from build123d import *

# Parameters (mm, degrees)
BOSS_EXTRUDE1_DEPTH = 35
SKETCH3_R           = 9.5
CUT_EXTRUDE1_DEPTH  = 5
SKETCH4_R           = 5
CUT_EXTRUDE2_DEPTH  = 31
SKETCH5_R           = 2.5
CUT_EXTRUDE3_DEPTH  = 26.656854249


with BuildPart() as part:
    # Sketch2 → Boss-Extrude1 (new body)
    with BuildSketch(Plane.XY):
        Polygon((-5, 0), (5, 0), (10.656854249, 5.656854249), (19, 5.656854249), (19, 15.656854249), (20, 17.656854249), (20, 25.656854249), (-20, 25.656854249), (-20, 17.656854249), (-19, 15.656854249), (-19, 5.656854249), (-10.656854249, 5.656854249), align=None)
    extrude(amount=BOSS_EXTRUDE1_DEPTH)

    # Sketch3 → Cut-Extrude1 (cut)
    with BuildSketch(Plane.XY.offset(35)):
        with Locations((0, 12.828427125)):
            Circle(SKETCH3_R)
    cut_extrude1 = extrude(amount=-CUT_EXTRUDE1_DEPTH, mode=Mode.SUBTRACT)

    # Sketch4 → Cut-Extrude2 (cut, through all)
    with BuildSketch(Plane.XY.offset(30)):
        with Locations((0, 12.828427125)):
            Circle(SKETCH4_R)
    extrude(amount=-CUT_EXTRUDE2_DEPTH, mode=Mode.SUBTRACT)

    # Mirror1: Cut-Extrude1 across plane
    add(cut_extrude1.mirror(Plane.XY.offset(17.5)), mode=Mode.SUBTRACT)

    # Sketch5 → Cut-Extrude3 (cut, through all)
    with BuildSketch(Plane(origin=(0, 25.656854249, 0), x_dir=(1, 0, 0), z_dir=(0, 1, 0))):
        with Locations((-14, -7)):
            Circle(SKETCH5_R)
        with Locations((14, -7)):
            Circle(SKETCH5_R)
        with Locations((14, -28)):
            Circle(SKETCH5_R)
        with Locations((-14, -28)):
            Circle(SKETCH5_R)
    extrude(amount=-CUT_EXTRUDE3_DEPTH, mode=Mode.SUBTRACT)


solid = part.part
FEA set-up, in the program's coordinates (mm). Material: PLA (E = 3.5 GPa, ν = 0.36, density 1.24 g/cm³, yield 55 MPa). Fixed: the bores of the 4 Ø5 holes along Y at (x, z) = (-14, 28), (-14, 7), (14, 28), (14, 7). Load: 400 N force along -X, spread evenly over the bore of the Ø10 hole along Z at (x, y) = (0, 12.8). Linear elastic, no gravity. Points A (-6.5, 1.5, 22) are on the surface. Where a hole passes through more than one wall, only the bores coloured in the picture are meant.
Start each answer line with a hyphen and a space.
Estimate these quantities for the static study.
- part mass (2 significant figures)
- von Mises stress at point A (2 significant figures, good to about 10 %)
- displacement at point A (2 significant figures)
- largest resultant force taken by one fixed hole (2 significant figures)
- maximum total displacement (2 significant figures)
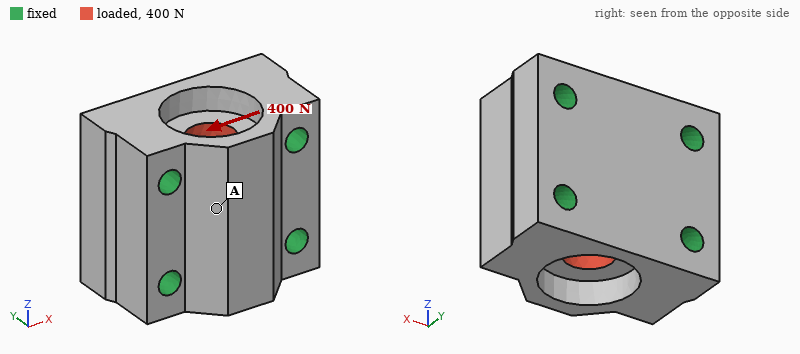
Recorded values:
- 30 g
- 0.17 MPa
- 1.4 µm
- 100 N
- 2.4 µm
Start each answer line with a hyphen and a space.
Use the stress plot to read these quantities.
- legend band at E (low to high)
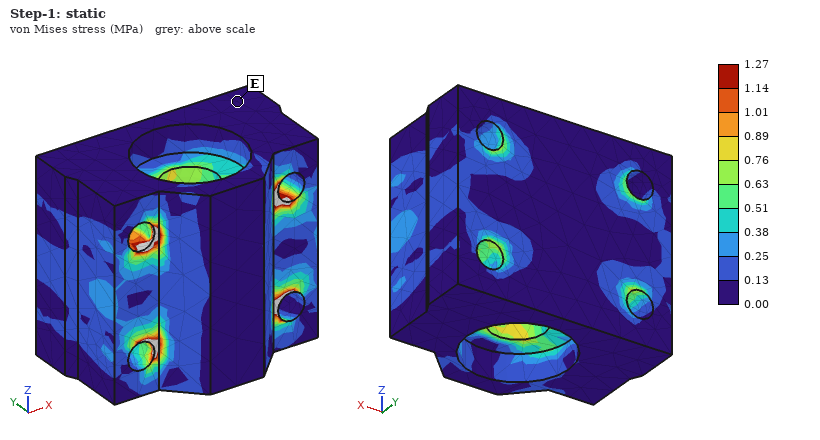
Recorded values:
- 0.00 to 0.13 MPa
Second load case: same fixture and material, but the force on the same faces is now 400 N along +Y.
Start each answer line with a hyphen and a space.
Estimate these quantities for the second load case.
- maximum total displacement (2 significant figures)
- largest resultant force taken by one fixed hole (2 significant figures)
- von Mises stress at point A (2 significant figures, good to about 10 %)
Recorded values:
- 4.4 µm
- 100 N
- 0.43 MPa
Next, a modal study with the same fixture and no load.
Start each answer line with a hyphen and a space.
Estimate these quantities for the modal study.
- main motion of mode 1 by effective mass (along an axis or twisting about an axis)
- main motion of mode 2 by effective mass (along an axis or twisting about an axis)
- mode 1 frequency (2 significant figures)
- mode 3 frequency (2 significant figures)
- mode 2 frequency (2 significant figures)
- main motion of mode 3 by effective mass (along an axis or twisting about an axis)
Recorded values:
- along Z
- along Y
- 15 kHz
- 19 kHz
- 16 kHz
- along Z
